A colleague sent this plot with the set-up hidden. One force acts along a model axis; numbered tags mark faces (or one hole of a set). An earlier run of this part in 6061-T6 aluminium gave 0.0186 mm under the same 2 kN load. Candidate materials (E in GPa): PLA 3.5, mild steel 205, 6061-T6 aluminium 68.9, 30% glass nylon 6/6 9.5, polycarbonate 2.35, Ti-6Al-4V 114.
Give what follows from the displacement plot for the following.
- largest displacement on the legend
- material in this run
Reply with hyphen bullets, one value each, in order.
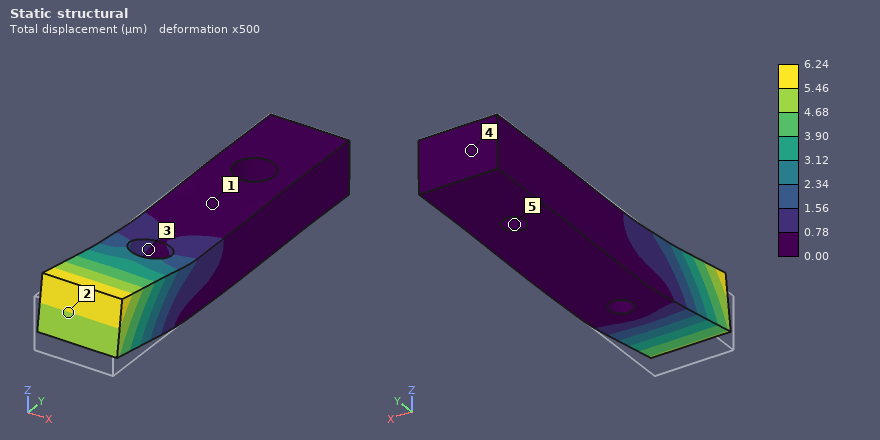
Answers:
- 6.24 µm
- mild steel
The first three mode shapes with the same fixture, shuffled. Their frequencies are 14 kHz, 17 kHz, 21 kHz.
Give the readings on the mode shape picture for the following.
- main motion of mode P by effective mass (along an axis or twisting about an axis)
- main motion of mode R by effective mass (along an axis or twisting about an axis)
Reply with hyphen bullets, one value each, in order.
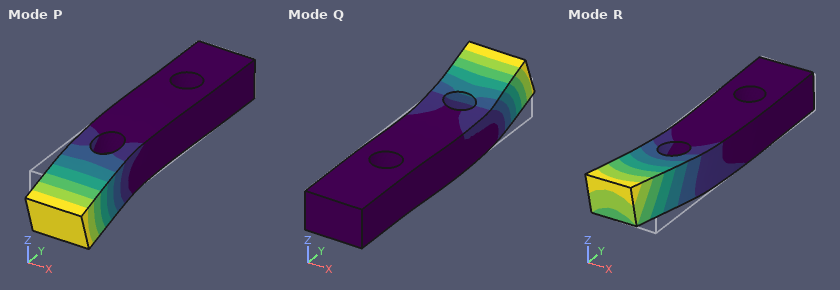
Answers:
- along Z
- along X
